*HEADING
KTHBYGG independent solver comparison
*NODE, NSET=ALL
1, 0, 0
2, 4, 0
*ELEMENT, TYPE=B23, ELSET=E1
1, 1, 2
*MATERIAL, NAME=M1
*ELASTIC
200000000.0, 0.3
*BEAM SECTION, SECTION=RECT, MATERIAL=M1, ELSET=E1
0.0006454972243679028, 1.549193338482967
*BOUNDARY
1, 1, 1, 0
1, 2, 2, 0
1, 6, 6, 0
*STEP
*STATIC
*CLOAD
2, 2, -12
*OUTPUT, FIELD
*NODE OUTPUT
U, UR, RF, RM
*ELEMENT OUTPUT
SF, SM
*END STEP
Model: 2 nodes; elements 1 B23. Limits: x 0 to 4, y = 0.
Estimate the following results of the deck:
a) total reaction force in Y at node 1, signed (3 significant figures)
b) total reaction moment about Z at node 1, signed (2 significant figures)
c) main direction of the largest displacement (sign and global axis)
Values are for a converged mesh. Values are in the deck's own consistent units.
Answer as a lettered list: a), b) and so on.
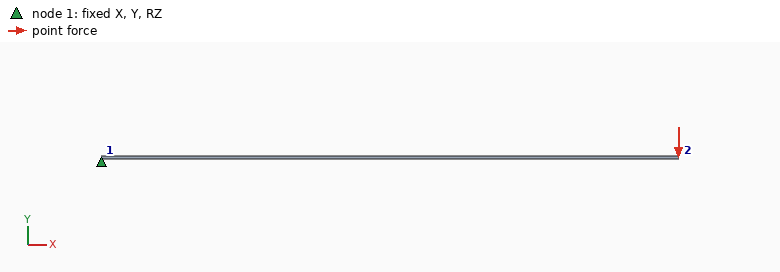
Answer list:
a) 12.0
b) 48
c) -Y
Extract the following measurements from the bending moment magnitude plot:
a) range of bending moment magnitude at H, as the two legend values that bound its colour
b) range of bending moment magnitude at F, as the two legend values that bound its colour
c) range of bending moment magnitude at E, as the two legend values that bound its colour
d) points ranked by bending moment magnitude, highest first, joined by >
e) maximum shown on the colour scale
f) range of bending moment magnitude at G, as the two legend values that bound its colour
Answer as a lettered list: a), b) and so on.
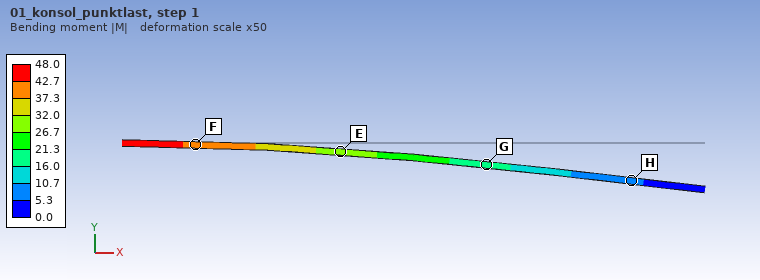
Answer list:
a) 5.3 to 10.7
b) 37.3 to 42.7
c) 26.7 to 32.0
d) F > E > G > H
e) 48.0
f) 16.0 to 21.3
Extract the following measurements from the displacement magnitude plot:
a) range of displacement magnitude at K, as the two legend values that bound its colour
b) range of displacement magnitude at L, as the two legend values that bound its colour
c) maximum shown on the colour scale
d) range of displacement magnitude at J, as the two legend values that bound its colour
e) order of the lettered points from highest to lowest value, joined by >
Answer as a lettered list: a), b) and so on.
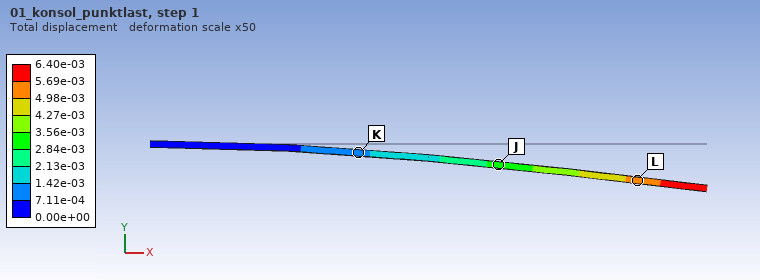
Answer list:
a) 7.11e-04 to 1.42e-03
b) 4.98e-03 to 5.69e-03
c) 6.40e-03
d) 2.84e-03 to 3.56e-03
e) L > J > K
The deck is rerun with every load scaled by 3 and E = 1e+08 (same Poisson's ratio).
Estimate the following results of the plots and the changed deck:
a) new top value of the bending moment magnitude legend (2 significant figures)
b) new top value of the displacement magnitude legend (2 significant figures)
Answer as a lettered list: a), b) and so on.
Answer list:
a) 140
b) 0.038
